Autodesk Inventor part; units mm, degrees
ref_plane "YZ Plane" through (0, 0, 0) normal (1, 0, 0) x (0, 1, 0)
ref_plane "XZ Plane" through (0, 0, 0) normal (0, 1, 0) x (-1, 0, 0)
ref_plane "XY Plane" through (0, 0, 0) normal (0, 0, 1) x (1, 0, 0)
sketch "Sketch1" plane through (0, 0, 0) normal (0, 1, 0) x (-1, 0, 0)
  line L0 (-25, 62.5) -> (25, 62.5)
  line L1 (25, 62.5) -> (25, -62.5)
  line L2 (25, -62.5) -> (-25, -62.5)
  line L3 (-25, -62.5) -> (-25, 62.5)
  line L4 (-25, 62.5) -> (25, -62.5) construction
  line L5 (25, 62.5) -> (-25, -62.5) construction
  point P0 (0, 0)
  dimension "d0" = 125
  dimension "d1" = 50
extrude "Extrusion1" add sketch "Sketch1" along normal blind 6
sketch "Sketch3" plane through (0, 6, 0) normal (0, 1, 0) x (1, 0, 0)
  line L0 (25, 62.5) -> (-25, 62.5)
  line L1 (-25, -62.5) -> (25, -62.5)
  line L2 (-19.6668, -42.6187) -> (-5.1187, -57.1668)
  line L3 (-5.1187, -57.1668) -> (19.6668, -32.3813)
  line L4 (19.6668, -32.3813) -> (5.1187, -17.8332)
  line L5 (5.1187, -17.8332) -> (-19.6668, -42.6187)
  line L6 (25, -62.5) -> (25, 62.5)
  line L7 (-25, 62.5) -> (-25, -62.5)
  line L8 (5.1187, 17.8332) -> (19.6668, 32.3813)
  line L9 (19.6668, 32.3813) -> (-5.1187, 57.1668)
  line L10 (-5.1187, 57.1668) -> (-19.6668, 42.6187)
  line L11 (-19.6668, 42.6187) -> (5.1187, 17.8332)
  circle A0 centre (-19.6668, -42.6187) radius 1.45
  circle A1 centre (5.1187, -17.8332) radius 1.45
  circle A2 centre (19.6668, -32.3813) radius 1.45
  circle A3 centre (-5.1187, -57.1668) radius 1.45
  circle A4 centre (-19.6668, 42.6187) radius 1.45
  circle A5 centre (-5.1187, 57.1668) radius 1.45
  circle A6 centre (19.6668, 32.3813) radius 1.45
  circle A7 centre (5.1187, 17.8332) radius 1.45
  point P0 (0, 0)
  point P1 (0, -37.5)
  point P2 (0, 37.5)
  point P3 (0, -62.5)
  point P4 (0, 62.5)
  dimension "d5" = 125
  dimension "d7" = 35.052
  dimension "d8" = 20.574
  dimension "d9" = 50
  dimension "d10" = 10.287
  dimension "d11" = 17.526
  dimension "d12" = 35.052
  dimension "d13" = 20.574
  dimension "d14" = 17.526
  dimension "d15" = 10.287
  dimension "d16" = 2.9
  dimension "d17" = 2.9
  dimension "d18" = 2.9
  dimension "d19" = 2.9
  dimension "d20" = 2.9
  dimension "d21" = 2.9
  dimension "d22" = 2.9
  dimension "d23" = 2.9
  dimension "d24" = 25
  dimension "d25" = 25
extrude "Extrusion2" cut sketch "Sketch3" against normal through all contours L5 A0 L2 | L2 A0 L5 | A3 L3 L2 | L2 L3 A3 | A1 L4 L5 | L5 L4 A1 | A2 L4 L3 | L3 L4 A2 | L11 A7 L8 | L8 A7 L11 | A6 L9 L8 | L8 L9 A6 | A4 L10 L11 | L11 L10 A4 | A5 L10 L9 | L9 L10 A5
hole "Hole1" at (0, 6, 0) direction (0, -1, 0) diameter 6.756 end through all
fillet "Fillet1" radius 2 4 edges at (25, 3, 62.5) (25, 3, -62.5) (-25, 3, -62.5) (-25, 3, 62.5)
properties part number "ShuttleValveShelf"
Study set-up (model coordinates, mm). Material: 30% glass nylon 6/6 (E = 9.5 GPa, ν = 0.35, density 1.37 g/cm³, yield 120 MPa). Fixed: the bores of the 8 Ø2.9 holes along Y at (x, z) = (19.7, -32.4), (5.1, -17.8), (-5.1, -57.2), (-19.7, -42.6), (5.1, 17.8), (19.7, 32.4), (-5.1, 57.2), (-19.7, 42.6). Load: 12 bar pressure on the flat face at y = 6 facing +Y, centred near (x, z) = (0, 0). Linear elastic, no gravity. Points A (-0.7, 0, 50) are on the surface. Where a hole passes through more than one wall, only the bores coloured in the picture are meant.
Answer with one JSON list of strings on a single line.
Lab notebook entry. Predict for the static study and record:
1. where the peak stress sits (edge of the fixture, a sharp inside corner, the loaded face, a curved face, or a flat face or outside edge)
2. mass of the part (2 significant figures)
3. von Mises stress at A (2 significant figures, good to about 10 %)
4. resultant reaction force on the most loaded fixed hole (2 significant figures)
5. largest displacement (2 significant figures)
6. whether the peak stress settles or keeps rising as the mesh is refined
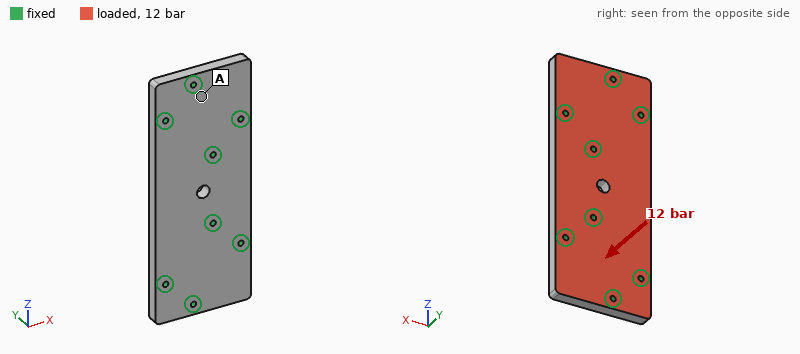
["edge of the fixture", "51 g", "13 MPa", "1.5 kN", "0.49 mm", "keeps rising"]
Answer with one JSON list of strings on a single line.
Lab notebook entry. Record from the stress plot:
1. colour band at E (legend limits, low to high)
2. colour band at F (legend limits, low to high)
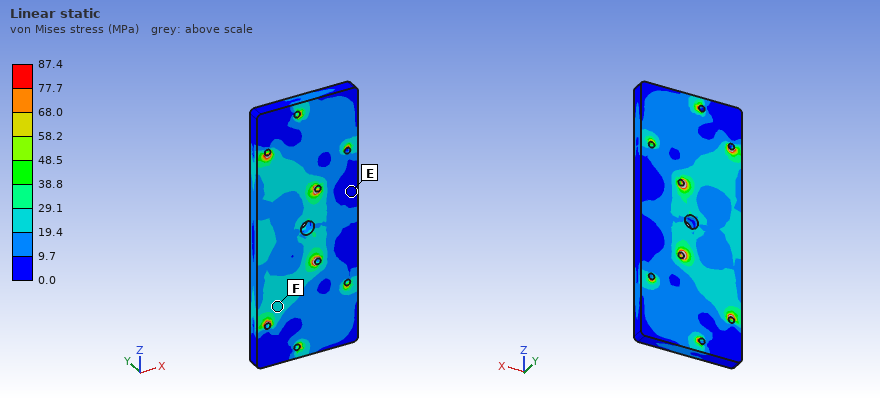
["0.0 to 9.7 MPa", "19.4 to 29.1 MPa"]
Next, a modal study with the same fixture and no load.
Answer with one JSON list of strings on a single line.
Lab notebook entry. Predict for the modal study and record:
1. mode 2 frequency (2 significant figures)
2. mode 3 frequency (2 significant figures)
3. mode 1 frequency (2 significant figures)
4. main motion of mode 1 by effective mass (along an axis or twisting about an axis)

["5100 Hz", "5100 Hz", "3600 Hz", "along Y"]
